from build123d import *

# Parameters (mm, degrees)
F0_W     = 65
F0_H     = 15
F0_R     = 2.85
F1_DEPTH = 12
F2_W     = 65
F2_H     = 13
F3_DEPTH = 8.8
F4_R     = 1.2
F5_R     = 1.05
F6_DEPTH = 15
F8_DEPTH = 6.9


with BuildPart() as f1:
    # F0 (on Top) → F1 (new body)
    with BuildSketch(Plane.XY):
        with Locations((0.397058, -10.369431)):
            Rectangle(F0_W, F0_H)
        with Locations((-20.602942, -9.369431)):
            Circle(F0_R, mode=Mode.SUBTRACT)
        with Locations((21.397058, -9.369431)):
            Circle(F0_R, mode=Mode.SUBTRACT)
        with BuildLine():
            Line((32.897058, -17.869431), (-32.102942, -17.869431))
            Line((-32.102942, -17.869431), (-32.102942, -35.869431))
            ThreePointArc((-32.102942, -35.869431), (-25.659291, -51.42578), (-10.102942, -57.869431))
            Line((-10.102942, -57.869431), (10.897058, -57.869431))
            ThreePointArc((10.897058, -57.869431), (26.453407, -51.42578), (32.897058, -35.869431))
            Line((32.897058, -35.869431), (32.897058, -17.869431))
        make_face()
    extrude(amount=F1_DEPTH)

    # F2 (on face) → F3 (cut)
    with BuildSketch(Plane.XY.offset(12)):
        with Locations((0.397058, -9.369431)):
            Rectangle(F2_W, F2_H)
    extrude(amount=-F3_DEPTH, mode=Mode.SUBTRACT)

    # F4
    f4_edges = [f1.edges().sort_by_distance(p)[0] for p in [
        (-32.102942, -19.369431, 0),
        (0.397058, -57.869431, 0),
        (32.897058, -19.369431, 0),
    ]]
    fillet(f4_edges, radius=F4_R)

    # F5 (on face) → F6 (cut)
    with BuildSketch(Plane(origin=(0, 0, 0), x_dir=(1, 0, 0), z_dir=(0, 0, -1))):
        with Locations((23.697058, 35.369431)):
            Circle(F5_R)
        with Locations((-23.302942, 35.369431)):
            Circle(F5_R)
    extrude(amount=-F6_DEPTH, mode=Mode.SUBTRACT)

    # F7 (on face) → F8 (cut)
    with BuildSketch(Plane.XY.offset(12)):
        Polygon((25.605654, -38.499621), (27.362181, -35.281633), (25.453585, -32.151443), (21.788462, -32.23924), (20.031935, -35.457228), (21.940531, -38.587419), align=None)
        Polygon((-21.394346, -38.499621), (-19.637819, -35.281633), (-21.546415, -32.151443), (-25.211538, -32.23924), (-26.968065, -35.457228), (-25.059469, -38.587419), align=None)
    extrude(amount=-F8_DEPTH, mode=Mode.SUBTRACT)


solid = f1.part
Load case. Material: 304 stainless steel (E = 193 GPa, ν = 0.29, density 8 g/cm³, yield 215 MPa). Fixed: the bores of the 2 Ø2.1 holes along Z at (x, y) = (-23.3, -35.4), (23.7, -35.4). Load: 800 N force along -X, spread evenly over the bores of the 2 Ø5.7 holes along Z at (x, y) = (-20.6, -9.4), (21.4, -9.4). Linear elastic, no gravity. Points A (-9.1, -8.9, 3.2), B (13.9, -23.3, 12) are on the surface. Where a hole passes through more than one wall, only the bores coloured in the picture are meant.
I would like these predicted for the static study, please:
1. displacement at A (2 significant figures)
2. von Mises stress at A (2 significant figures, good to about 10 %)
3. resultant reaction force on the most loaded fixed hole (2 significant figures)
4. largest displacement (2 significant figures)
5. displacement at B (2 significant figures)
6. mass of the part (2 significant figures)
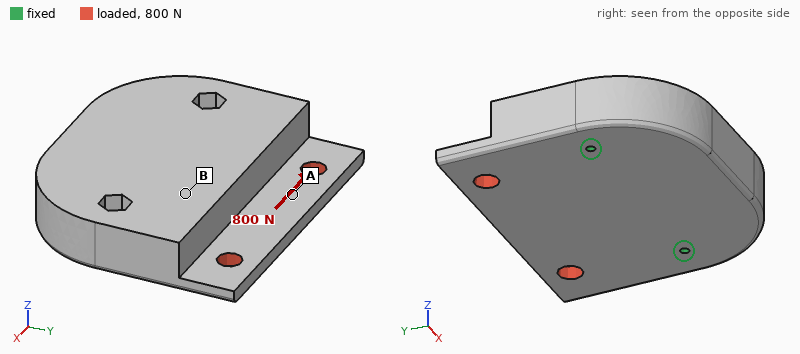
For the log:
1.4 µm
5.4 MPa
590 N
2.4 µm
0.60 µm
260 g
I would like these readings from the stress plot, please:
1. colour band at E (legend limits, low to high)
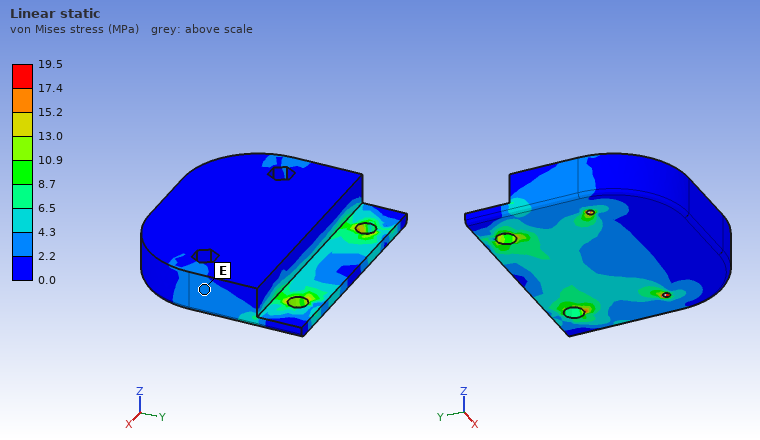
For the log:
2.2 to 4.3 MPa
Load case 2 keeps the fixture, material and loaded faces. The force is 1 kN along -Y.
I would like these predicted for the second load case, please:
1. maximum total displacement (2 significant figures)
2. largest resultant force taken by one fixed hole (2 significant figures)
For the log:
3.4 µm
510 N
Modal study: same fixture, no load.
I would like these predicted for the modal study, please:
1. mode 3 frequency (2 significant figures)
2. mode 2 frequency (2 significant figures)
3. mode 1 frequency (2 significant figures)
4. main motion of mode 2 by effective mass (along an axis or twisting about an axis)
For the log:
9400 Hz
8700 Hz
2900 Hz
along Z
